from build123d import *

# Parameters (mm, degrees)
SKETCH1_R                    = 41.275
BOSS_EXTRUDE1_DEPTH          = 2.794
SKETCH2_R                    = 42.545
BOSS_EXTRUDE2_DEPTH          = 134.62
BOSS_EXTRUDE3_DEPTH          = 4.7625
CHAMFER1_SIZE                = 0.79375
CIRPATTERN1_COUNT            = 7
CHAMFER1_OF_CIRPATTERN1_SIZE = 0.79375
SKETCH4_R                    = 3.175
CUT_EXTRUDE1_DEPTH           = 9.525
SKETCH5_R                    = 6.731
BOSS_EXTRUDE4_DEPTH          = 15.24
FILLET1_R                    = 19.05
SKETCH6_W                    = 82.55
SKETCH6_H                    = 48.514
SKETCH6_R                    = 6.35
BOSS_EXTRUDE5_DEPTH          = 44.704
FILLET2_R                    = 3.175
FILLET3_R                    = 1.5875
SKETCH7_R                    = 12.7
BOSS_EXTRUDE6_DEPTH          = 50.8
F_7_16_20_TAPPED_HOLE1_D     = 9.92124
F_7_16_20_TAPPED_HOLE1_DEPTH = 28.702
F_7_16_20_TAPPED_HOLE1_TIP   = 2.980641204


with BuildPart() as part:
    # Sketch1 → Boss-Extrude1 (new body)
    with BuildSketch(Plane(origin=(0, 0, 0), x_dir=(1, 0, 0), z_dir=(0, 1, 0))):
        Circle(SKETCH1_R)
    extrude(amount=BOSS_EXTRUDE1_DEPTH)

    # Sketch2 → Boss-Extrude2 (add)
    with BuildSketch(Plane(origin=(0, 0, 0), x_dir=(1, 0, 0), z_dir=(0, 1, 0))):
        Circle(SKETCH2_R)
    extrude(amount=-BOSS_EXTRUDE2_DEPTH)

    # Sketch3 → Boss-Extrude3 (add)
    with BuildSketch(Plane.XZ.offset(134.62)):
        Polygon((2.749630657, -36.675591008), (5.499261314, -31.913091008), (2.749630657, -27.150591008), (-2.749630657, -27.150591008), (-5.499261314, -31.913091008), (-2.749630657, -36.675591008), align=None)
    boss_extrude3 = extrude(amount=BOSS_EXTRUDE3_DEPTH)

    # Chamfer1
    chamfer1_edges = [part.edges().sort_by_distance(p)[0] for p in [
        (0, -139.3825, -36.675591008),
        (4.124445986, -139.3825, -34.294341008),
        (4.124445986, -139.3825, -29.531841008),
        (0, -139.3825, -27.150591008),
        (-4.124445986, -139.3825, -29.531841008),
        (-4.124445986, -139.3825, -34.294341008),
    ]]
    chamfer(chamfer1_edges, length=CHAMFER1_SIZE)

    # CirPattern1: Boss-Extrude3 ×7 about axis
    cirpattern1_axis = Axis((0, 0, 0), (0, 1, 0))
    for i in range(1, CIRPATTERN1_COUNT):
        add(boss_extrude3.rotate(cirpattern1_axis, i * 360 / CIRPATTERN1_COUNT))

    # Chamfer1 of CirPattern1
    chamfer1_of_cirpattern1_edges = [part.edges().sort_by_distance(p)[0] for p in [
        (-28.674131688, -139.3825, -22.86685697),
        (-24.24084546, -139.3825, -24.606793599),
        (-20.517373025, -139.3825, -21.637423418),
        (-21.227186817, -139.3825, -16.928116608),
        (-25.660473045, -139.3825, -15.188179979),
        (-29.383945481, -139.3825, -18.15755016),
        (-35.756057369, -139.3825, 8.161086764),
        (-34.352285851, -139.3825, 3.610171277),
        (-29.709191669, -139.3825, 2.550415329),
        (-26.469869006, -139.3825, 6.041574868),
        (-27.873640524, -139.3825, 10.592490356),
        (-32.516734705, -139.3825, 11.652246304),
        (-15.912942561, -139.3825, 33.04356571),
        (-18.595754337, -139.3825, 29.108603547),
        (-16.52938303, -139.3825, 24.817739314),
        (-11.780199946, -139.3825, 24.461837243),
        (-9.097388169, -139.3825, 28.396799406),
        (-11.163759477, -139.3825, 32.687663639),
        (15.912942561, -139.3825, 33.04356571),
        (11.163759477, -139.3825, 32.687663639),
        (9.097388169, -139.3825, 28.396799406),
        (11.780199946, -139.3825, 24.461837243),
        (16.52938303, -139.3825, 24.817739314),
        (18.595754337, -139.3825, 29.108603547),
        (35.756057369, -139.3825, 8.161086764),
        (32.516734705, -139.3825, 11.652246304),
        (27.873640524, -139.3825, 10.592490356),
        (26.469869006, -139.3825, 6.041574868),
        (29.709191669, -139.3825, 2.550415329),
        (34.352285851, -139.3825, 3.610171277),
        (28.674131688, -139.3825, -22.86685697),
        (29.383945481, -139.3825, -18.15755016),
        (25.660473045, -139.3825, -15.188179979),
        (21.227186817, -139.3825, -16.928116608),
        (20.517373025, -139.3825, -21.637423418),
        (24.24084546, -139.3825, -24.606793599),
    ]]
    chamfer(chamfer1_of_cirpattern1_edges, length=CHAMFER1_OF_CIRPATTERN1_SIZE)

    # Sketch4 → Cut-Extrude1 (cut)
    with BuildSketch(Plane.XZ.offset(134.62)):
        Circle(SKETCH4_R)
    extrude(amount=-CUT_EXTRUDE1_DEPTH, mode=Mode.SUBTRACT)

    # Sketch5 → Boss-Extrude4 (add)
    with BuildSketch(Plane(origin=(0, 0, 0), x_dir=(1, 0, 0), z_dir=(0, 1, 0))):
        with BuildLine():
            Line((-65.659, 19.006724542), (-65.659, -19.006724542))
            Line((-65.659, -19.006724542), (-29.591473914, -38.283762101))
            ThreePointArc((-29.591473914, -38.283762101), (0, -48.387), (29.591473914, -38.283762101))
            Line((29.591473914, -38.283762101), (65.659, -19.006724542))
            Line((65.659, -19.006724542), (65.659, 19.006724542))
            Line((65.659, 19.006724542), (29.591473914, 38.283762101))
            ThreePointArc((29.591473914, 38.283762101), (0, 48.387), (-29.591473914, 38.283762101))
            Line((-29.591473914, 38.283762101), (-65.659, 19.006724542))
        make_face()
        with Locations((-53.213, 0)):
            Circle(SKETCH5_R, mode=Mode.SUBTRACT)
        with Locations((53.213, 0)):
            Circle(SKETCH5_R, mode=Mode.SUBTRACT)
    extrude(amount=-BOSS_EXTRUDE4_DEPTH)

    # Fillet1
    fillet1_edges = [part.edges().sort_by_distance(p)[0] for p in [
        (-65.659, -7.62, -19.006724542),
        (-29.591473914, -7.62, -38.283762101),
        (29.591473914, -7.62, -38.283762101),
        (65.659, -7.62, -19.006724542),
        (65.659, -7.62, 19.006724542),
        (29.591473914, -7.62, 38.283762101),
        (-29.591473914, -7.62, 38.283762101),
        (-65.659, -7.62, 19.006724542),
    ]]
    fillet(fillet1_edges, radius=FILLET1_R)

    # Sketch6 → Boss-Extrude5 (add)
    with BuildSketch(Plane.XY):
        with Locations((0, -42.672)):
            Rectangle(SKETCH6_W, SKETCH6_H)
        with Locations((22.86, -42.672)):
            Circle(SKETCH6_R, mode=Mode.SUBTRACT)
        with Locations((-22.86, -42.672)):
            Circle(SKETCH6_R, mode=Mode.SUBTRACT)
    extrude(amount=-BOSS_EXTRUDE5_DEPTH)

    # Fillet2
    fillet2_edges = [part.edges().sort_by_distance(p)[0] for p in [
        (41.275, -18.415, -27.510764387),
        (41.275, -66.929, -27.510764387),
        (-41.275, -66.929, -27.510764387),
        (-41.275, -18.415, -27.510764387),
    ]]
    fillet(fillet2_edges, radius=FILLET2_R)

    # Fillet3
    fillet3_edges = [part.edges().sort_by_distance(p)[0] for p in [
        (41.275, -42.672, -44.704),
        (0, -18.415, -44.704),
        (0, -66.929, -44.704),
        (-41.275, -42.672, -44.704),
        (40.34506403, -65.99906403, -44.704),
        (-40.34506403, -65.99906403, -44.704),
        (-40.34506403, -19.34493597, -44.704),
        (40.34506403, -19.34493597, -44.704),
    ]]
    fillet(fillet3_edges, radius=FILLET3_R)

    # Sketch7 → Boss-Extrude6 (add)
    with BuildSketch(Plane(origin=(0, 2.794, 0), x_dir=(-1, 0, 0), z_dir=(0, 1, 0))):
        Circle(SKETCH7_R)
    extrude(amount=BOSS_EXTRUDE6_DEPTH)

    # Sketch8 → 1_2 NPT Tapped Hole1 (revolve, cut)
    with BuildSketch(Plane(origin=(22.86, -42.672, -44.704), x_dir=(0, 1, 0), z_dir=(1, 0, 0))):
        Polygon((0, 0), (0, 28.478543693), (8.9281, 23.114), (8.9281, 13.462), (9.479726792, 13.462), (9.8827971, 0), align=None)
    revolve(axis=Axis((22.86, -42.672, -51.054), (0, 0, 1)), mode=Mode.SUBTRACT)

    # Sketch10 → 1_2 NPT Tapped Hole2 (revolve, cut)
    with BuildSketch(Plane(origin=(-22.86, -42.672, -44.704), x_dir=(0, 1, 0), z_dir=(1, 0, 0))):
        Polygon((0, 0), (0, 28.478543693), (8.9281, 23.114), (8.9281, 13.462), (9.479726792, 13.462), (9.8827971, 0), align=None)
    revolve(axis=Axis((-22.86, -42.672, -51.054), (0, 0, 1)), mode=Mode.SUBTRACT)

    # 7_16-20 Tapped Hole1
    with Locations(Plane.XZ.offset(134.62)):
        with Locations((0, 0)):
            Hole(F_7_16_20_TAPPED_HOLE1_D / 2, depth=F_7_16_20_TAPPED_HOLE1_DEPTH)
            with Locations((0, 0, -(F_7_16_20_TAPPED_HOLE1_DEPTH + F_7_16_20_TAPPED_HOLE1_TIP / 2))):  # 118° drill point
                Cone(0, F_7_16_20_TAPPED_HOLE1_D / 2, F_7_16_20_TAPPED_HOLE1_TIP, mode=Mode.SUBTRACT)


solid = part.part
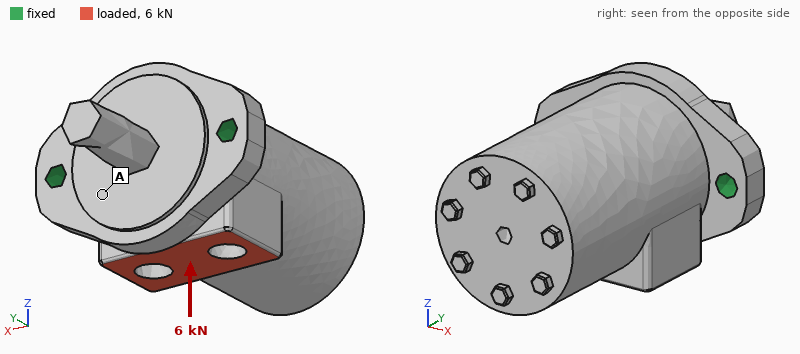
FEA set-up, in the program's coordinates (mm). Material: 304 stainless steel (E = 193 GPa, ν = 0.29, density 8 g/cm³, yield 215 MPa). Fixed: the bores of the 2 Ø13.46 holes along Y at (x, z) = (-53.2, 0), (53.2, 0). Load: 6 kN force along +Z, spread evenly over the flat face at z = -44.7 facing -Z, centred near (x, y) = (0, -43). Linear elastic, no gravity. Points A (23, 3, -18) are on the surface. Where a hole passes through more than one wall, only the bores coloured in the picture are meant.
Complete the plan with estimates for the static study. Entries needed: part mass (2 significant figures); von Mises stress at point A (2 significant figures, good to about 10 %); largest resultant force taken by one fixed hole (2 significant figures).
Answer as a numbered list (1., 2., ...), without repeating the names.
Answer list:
1. 7.1 kg
2. 6.6 MPa
3. 3.0 kN
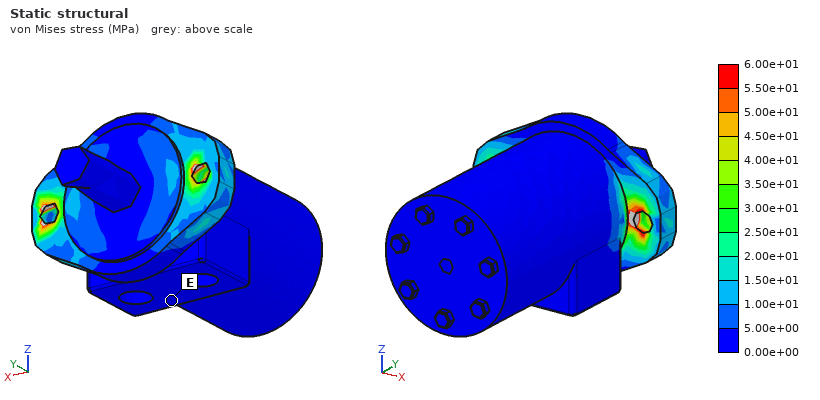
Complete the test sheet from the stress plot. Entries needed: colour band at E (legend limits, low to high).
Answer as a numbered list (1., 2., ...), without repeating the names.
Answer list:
1. 0.00e+00 to 5.00e+00 MPa
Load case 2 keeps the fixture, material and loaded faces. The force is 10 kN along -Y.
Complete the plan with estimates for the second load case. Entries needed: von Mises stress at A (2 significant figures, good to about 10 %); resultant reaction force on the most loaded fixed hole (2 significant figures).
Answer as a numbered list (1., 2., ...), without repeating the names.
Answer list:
1. 17 MPa
2. 5.3 kN
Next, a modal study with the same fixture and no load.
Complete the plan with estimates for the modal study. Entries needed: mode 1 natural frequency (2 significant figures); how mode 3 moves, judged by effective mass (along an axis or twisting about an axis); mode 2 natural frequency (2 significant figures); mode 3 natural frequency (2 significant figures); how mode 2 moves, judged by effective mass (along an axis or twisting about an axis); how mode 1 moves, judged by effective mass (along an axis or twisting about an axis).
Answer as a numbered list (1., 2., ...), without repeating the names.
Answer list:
1. 630 Hz
2. along Y
3. 2000 Hz
4. 3400 Hz
5. along X
6. along Z
